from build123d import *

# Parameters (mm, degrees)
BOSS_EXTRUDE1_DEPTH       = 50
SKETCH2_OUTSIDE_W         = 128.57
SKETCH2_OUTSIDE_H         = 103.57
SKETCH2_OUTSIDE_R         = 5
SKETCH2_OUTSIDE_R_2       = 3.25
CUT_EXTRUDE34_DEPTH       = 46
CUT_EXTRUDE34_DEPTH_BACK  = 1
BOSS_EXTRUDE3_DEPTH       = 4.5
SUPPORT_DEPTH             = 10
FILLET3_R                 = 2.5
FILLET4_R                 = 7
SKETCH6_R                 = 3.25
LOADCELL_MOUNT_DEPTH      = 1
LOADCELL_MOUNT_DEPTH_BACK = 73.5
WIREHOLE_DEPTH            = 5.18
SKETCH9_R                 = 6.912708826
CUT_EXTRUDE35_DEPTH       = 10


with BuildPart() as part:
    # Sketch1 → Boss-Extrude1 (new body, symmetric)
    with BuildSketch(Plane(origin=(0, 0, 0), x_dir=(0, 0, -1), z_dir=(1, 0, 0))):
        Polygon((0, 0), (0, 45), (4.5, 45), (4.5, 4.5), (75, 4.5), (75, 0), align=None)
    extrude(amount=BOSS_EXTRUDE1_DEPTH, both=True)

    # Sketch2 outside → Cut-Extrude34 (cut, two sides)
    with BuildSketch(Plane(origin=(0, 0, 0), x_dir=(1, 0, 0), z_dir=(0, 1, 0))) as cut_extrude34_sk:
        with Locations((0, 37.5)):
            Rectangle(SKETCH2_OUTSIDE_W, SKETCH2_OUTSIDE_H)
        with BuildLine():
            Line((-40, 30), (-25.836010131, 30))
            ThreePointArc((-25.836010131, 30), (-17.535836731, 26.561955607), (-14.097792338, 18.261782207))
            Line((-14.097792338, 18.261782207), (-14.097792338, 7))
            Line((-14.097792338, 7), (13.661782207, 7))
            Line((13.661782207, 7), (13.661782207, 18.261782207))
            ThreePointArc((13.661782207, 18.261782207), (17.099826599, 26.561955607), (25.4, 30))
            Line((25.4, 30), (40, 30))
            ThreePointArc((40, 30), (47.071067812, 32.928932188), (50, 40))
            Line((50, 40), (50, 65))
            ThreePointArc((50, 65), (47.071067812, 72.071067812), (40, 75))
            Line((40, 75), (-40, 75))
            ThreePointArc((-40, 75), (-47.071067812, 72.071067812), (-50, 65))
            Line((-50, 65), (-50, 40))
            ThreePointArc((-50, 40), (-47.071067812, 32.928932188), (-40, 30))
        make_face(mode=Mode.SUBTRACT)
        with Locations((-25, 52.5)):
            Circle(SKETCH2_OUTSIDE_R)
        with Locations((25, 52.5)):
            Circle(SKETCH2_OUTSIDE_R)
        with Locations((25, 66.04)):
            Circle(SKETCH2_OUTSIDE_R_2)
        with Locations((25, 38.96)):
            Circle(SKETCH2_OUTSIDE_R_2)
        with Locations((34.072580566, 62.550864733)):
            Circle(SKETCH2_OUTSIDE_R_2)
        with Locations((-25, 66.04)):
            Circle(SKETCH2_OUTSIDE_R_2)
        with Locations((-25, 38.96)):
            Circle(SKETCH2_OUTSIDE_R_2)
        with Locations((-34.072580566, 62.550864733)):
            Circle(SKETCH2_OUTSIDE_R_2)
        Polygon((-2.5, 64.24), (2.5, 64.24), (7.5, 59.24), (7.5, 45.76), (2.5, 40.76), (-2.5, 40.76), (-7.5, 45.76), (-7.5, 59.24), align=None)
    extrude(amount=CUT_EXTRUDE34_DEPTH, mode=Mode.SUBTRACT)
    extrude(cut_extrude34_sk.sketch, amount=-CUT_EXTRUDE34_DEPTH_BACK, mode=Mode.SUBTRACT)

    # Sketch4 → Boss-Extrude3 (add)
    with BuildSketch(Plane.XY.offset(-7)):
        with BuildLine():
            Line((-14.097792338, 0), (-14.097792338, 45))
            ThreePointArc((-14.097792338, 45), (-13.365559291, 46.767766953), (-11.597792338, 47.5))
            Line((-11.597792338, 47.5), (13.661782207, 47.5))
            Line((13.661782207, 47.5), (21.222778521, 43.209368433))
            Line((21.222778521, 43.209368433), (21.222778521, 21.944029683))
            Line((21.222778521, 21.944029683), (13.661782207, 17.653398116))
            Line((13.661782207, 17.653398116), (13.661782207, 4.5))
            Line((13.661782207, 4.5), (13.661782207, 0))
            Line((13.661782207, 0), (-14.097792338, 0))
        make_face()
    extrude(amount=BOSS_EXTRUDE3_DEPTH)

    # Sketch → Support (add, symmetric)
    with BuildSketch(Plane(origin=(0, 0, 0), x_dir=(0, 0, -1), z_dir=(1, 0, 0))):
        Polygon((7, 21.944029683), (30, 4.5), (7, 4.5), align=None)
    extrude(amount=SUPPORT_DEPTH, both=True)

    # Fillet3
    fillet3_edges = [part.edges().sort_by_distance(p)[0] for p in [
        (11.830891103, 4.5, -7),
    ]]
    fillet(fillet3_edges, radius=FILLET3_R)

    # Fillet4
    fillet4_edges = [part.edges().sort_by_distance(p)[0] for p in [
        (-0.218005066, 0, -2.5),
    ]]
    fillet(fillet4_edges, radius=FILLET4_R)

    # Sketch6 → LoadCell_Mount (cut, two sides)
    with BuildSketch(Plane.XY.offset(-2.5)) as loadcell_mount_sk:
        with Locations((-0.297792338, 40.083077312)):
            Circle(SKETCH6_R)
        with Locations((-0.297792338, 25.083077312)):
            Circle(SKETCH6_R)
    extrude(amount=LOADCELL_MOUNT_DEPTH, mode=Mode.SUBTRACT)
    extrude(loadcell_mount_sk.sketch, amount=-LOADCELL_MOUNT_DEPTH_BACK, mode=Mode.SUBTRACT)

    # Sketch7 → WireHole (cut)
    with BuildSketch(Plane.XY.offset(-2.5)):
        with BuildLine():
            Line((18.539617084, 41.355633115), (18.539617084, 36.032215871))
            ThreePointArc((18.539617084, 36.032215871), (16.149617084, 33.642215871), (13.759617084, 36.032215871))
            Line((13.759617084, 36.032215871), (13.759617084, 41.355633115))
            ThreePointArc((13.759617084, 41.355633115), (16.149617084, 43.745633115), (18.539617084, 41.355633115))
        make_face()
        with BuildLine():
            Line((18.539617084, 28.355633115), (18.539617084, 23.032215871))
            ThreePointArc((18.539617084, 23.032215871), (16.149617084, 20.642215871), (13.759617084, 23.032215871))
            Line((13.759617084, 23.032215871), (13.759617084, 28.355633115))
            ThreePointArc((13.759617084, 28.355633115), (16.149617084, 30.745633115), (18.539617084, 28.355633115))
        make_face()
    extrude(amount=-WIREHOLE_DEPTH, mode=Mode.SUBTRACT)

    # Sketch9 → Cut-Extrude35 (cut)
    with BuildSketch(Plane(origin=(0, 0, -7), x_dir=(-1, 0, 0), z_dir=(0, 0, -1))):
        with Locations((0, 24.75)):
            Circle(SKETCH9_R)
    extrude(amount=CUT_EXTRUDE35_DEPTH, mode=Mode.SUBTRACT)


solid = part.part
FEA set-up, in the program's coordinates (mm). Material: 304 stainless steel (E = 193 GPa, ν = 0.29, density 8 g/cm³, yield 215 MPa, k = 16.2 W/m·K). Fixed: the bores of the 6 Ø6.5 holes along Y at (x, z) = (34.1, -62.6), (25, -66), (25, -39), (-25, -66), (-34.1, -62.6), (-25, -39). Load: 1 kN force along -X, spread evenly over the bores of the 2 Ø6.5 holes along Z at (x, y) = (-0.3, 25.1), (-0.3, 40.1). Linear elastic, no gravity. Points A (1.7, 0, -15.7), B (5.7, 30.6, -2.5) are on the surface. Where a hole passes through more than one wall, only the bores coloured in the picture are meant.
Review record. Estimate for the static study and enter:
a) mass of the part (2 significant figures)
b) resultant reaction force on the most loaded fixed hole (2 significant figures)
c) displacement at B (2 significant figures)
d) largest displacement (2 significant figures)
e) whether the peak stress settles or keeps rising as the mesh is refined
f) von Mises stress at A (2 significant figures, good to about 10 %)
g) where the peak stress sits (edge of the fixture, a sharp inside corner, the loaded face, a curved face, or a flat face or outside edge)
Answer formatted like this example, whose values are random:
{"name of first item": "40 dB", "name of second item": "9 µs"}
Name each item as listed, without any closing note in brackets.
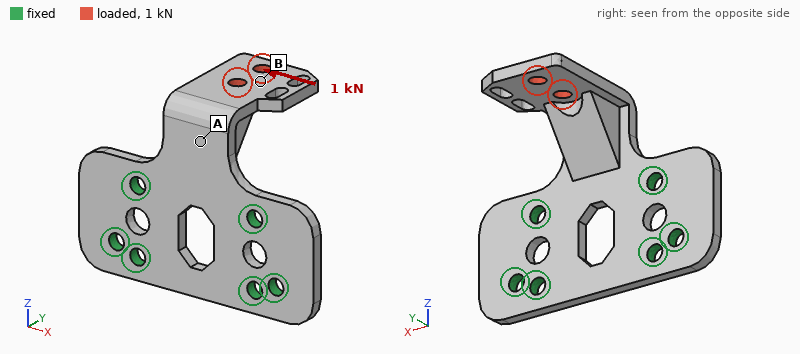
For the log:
{"mass of the part": "240 g", "resultant reaction force on the most loaded fixed hole": "1.2 kN", "displacement at B": "0.077 mm", "largest displacement": "0.13 mm", "whether the peak stress settles or keeps rising as the mesh is refined": "keeps rising", "von Mises stress at A": "38 MPa", "where the peak stress sits": "edge of the fixture"}
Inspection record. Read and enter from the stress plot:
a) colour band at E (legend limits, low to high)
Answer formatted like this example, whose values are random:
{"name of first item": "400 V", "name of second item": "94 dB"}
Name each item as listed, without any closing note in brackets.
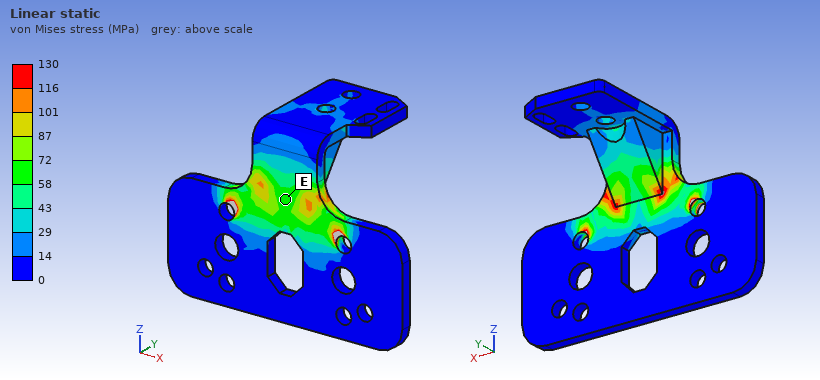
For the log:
{"colour band at E": "58 to 72 MPa"}
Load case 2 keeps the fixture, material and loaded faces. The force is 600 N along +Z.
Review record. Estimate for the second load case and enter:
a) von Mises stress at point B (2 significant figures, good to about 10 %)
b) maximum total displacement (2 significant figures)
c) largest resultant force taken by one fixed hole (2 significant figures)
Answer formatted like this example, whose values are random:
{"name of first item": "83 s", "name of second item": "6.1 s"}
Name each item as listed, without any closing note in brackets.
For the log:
{"von Mises stress at point B": "29 MPa", "maximum total displacement": "0.33 mm", "largest resultant force taken by one fixed hole": "230 N"}
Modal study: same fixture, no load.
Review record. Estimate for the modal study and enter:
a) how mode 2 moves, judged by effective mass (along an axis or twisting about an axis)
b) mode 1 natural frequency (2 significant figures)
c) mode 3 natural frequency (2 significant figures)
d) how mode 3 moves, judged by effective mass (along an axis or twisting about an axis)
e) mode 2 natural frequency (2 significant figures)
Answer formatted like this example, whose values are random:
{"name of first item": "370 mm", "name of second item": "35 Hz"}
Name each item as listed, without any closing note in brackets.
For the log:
{"how mode 2 moves, judged by effective mass": "along X", "mode 1 natural frequency": "990 Hz", "mode 3 natural frequency": "3700 Hz", "how mode 3 moves, judged by effective mass": "along Y", "mode 2 natural frequency": "2700 Hz"}
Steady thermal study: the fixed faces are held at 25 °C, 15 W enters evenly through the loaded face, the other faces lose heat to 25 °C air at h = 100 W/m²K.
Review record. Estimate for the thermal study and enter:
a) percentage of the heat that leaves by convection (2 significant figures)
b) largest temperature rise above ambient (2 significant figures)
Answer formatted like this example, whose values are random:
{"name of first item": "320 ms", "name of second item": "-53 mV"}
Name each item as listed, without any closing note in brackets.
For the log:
{"percentage of the heat that leaves by convection": "95 %", "largest temperature rise above ambient": "72 K"}
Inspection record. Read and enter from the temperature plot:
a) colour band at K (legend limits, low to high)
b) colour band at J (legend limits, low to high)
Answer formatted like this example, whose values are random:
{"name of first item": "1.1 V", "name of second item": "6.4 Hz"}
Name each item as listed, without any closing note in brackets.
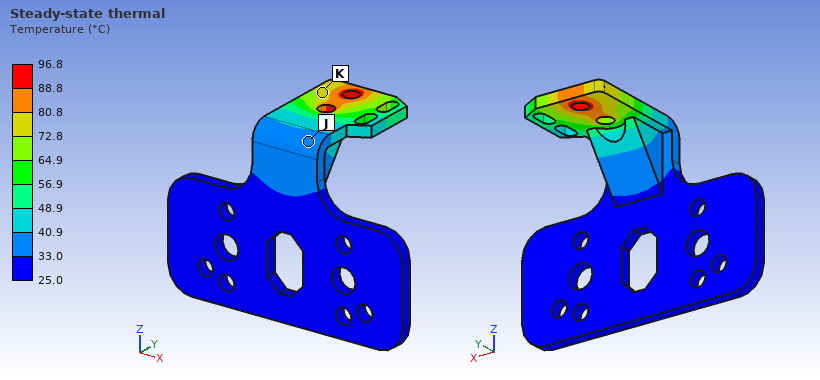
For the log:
{"colour band at K": "72.8 to 80.8 °C", "colour band at J": "33.0 to 40.9 °C"}
